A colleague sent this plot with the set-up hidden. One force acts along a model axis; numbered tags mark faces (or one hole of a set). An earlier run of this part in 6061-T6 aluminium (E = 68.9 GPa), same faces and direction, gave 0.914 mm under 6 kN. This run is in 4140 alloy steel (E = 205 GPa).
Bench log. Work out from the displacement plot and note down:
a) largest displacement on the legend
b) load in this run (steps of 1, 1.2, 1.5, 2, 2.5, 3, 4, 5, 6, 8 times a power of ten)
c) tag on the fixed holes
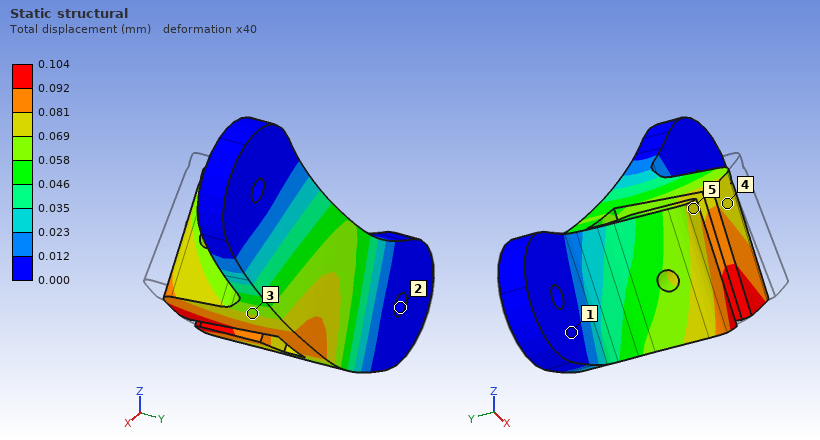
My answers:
0.104 mm
2 kN
2
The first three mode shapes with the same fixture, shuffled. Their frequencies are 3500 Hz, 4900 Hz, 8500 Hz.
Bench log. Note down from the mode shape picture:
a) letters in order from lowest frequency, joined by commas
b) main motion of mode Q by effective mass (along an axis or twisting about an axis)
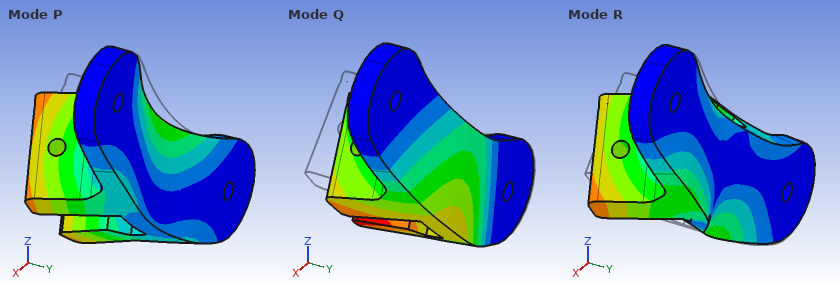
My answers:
Q, P, R
along Y
